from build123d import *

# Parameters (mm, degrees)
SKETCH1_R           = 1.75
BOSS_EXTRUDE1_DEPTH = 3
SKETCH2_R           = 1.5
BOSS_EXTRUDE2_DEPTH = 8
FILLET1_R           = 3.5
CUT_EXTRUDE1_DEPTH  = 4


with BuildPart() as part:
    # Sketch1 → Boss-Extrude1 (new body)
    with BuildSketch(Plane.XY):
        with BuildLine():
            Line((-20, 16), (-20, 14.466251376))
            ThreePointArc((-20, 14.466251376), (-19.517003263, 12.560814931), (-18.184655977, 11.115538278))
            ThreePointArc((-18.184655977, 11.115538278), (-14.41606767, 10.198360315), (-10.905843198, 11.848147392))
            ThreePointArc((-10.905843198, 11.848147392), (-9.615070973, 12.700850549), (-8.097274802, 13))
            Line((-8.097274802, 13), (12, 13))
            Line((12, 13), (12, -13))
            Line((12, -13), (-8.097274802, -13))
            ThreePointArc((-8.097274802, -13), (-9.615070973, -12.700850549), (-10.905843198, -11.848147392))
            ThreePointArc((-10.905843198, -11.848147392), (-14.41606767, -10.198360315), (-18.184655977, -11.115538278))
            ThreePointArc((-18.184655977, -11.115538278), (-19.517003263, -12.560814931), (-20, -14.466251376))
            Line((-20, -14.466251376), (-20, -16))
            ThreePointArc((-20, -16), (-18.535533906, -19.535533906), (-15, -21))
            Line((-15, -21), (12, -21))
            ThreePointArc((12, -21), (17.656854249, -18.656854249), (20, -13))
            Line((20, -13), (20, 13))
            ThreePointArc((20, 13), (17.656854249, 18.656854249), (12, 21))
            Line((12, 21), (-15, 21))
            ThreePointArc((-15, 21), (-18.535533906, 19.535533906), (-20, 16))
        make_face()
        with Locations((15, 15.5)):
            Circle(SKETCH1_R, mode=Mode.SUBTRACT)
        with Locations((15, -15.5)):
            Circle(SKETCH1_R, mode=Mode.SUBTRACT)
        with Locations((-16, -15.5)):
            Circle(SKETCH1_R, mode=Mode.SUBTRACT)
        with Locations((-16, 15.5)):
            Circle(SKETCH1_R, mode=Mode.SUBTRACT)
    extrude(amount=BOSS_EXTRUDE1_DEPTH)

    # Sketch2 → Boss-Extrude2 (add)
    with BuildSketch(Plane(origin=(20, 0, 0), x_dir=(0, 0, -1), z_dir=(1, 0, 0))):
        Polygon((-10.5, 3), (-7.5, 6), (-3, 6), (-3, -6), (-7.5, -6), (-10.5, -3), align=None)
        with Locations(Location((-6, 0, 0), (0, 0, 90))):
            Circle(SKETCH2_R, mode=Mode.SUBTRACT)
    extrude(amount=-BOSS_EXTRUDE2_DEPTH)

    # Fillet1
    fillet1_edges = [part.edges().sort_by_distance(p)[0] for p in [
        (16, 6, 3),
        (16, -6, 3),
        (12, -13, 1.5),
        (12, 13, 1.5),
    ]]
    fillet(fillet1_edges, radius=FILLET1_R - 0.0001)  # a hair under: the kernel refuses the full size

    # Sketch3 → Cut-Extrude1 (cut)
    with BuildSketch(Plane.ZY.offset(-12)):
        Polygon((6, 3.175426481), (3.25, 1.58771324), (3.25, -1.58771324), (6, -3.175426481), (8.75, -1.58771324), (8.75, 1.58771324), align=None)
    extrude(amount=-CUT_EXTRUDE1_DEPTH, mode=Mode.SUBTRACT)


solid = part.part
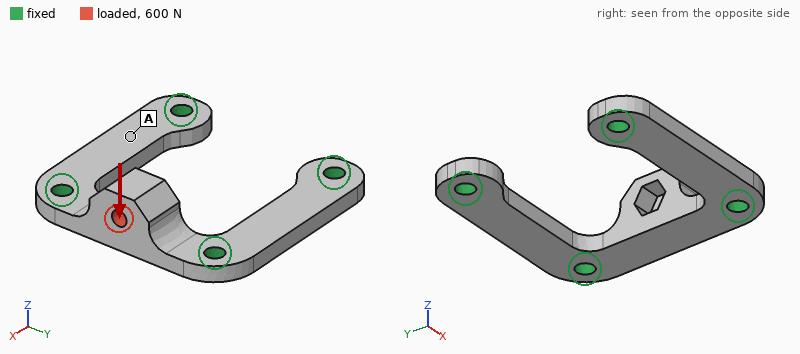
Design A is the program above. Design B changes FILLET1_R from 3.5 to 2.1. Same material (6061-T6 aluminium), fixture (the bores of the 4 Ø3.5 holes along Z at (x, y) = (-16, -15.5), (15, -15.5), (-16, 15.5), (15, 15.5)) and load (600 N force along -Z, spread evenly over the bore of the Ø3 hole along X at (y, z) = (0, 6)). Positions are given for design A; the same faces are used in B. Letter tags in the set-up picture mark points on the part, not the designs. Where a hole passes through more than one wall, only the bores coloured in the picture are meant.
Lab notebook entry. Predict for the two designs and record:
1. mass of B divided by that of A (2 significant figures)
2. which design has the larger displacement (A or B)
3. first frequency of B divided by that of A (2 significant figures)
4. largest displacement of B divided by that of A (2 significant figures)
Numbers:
0.99
B
0.94
1.1
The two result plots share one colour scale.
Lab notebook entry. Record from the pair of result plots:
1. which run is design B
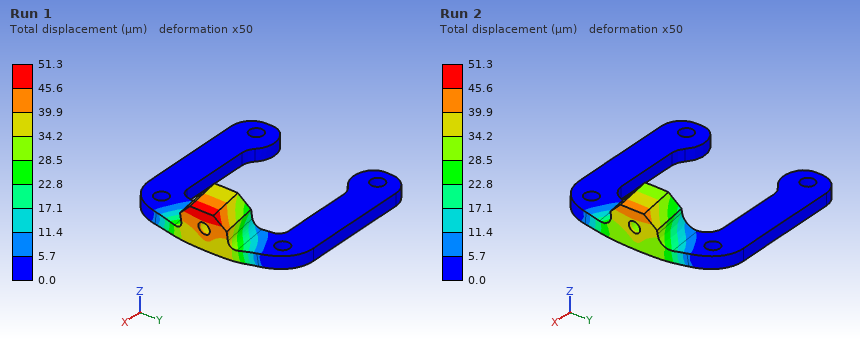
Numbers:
Run 1
